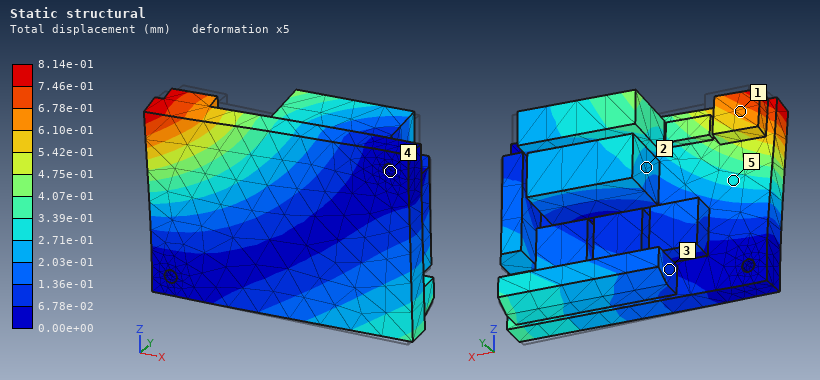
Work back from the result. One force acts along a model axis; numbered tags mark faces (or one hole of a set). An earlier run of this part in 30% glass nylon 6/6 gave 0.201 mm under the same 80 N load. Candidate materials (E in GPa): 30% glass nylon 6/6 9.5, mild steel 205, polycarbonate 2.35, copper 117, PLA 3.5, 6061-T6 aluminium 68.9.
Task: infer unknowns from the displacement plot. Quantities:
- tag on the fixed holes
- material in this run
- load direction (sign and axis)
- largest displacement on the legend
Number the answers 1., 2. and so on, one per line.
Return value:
1. 4
2. polycarbonate
3. -Y
4. 8.14e-01 mm
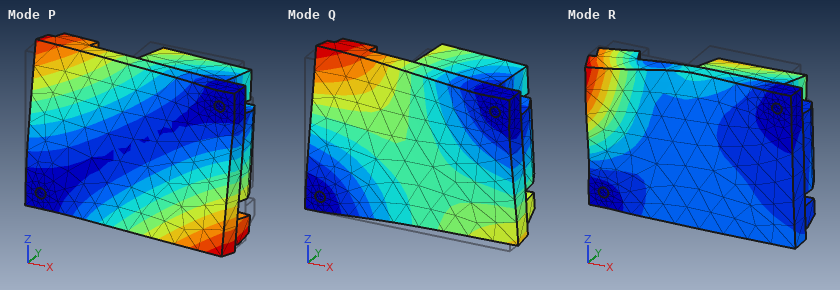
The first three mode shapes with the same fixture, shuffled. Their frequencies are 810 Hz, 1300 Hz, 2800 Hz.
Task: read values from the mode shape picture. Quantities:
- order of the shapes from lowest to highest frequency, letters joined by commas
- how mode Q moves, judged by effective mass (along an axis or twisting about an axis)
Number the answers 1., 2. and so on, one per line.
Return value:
1. P, Q, R
2. along Y
